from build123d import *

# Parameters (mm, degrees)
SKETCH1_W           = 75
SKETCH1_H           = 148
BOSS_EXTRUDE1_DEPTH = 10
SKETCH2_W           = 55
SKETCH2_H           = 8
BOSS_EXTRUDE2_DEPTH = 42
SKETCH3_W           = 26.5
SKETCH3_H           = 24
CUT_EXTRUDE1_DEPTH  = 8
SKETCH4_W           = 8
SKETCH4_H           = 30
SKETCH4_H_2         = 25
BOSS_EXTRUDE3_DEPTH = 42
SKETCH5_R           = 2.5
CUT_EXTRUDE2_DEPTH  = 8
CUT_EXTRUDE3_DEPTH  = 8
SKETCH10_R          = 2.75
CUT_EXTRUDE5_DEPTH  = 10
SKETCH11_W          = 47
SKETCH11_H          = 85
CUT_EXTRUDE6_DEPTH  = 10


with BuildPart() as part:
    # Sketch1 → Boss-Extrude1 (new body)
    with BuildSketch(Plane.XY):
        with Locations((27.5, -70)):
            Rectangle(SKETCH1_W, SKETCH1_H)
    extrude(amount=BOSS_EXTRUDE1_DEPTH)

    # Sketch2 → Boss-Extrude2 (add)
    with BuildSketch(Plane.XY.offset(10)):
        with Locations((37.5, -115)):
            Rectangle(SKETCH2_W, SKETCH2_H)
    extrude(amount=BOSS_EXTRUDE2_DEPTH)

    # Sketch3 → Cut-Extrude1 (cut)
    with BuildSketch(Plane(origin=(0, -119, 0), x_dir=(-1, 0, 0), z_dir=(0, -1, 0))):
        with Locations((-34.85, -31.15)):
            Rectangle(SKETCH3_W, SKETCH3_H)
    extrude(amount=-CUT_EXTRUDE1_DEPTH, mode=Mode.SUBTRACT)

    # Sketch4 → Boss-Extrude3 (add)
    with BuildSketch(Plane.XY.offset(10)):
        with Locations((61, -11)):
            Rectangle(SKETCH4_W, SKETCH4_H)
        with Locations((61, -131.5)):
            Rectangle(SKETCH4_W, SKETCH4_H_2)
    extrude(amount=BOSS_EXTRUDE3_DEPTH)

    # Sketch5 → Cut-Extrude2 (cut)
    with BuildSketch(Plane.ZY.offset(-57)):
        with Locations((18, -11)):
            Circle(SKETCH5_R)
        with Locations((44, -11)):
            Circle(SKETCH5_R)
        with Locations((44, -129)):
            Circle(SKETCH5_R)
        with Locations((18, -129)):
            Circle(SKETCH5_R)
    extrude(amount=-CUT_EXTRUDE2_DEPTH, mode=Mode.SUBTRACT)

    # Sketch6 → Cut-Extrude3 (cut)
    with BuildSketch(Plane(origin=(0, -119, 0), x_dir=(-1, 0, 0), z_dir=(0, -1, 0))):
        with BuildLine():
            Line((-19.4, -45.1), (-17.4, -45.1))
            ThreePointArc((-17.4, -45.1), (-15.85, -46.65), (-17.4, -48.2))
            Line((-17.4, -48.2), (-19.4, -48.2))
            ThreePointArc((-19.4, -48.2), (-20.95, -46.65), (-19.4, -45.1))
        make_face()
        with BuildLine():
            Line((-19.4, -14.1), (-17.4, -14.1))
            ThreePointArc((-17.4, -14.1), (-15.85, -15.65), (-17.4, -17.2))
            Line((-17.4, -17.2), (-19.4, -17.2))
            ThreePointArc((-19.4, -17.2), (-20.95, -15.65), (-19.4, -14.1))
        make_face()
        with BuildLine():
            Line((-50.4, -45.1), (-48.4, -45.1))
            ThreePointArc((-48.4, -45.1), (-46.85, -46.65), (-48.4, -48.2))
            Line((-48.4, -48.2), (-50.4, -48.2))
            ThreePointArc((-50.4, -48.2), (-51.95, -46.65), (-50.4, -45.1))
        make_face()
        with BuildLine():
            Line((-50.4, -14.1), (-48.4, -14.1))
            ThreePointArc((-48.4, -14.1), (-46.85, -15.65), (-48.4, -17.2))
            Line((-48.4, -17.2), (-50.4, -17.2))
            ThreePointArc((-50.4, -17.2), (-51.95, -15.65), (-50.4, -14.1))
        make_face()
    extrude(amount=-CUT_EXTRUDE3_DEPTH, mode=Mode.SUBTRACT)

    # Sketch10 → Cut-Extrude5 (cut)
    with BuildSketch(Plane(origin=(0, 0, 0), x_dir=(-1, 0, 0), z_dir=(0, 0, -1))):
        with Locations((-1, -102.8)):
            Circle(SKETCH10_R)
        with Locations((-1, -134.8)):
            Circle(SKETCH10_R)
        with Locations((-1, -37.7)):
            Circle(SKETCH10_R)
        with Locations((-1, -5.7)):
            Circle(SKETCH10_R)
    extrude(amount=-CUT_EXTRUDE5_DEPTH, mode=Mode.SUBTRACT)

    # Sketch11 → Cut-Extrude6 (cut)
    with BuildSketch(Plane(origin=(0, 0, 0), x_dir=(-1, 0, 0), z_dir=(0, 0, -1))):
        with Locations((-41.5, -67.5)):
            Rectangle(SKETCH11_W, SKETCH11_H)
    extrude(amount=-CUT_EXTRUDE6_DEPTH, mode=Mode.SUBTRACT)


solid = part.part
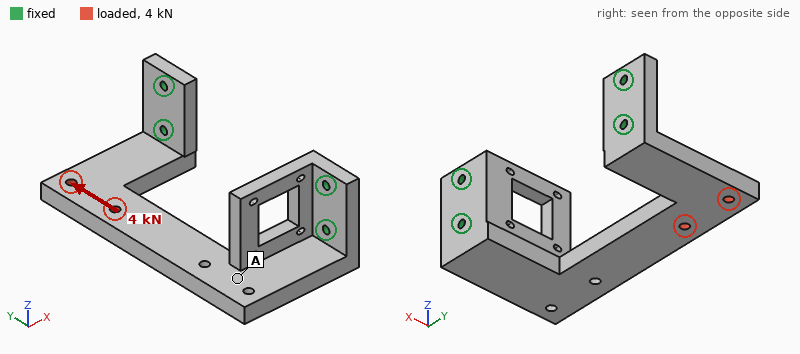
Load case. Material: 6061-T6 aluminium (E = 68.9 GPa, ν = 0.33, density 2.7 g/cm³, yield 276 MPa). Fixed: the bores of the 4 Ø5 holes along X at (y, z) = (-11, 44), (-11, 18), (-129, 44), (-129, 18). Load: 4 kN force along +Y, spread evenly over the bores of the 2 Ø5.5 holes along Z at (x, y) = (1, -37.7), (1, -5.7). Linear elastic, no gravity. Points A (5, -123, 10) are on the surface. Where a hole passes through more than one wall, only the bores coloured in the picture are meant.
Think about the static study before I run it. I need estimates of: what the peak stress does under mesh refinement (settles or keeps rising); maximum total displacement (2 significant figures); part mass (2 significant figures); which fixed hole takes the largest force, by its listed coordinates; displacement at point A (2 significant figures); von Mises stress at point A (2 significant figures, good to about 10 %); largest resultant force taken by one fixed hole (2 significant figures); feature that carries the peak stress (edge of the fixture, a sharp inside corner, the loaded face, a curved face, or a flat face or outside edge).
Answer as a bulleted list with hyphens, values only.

- keeps rising
- 0.17 mm
- 270 g
- (-129, 18)
- 0.12 mm
- 15 MPa
- 3.5 kN
- edge of the fixture
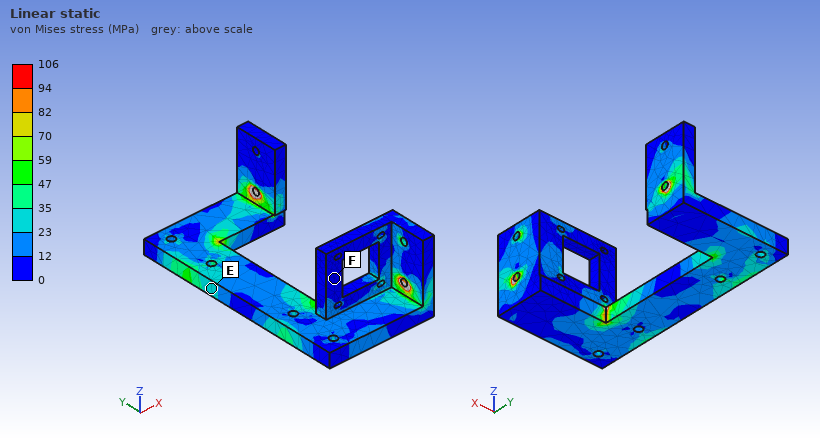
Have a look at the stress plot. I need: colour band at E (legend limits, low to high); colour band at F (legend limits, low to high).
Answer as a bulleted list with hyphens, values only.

- 23 to 35 MPa
- 0 to 12 MPa
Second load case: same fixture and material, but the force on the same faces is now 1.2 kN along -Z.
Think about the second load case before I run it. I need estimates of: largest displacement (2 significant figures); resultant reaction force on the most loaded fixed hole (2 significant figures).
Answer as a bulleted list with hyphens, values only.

- 0.68 mm
- 1.3 kN
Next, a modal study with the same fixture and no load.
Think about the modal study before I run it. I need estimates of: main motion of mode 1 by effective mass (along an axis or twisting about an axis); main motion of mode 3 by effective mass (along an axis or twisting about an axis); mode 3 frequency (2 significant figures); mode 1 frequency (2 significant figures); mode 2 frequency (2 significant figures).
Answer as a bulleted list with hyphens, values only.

- along Z
- along Y
- 2500 Hz
- 1100 Hz
- 1900 Hz
